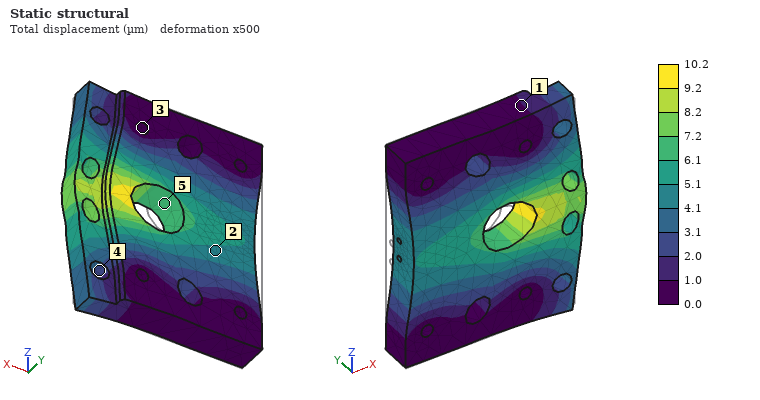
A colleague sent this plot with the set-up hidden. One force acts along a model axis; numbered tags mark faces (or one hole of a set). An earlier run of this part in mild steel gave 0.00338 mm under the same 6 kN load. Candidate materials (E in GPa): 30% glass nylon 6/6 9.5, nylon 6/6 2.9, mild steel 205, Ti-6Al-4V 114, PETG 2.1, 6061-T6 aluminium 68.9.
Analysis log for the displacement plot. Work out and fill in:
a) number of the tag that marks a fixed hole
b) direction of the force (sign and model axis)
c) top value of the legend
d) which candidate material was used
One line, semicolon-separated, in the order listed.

3; +X; 10.2 µm; 6061-T6 aluminium
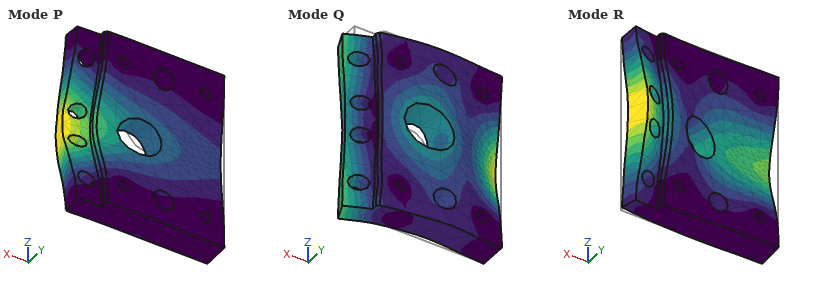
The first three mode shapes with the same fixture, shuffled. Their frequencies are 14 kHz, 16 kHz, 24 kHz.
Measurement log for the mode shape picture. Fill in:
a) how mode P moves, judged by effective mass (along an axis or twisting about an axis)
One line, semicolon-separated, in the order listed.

along Y
